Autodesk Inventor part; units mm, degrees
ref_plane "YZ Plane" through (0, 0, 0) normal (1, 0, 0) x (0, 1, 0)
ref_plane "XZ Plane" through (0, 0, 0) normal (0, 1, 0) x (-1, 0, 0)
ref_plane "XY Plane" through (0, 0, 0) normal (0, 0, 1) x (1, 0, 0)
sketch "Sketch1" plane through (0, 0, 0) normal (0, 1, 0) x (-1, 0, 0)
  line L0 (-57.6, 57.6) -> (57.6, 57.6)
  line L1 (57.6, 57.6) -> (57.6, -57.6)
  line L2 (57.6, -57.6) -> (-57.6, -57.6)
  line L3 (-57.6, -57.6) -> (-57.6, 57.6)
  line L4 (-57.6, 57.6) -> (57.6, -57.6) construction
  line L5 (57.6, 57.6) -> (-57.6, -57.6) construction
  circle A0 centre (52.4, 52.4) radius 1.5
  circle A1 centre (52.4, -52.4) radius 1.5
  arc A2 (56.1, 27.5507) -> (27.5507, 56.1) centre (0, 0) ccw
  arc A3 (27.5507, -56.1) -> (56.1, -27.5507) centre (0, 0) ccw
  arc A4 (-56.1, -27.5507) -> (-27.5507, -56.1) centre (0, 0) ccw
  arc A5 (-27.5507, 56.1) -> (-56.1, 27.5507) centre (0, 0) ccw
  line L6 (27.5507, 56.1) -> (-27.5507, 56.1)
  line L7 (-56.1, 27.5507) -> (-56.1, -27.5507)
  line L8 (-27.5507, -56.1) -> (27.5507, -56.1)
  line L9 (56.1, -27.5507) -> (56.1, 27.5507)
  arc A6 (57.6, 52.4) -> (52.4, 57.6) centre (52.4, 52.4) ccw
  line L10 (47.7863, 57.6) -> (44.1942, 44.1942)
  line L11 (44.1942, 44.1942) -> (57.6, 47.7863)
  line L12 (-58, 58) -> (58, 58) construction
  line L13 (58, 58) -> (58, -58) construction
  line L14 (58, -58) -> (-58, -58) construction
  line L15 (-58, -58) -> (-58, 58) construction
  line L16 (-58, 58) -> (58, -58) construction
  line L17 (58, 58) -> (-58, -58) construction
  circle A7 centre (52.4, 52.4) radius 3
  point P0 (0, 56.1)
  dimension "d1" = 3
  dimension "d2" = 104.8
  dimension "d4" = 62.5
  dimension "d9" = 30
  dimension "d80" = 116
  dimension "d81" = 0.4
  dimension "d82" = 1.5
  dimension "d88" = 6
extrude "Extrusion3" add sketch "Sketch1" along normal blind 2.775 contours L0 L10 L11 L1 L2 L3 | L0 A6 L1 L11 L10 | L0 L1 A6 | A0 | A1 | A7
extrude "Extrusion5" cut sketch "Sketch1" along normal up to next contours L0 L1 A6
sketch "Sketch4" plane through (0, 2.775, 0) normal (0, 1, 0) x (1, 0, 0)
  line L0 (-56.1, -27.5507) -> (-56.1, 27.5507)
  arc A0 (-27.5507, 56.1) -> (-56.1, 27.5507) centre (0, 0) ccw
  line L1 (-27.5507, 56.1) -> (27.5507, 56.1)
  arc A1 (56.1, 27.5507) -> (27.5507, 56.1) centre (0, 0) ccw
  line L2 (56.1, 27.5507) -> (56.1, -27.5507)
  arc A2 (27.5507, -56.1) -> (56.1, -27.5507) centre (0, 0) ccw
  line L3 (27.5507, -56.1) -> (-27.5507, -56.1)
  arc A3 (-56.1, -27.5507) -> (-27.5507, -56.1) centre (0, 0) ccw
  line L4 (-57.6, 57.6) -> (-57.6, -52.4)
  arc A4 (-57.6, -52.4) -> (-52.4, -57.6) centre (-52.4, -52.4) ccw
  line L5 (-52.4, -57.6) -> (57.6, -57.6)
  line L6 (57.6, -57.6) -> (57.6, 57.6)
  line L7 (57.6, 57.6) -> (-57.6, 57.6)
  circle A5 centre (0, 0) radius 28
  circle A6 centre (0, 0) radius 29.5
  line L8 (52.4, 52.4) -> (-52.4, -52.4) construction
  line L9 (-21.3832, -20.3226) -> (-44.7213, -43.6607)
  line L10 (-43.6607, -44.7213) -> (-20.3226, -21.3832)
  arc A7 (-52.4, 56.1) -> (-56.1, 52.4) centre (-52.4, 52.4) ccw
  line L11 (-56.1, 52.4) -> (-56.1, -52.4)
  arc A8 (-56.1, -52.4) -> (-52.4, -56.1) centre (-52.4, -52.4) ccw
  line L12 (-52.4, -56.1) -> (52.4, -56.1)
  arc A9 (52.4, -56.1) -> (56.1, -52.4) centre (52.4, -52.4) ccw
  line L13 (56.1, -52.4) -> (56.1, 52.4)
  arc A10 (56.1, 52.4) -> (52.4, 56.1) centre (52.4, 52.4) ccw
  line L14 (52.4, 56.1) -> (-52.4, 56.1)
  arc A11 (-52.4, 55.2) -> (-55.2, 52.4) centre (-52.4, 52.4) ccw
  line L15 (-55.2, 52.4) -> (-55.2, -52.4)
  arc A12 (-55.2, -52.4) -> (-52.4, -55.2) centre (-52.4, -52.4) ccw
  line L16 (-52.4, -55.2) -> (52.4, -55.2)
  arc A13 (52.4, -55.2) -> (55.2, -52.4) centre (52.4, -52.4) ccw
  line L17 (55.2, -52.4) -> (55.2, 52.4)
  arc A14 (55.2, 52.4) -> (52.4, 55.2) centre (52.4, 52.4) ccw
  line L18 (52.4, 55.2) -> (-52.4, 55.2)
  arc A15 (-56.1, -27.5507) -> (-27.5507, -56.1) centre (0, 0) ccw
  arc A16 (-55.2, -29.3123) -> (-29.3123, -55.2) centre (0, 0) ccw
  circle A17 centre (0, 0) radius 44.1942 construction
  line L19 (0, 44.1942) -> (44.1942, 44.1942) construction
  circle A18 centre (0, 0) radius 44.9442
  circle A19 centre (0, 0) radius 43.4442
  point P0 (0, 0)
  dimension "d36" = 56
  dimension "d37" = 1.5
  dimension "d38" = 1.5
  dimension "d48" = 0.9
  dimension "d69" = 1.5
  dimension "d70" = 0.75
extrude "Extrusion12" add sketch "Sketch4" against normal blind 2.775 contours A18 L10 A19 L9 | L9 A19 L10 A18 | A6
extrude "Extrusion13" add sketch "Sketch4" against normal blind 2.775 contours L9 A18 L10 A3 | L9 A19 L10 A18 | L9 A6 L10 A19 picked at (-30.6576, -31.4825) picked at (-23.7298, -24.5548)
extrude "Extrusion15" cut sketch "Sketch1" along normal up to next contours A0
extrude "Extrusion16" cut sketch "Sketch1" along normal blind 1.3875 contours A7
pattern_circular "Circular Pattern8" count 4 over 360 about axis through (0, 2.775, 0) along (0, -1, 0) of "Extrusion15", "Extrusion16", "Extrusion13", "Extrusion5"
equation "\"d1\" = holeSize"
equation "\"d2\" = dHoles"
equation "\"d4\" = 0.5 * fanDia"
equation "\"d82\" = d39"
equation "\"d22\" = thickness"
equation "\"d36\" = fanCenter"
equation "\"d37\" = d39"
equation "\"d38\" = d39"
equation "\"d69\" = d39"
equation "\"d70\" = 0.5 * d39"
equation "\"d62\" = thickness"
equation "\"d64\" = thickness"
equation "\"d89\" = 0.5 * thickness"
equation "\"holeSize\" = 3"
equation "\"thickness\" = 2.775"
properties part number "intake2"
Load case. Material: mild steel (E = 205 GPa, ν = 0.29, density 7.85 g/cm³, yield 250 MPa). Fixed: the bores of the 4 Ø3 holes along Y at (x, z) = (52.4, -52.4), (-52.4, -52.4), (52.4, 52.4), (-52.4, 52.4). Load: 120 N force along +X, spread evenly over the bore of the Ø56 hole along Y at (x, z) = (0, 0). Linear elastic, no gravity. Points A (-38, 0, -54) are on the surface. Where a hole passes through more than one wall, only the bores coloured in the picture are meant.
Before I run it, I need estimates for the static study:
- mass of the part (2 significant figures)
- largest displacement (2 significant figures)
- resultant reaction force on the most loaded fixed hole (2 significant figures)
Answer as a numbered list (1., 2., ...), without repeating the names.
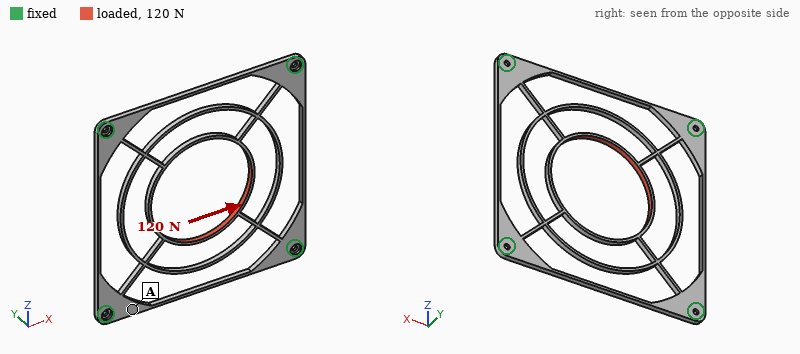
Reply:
1. 60 g
2. 0.18 mm
3. 39 N
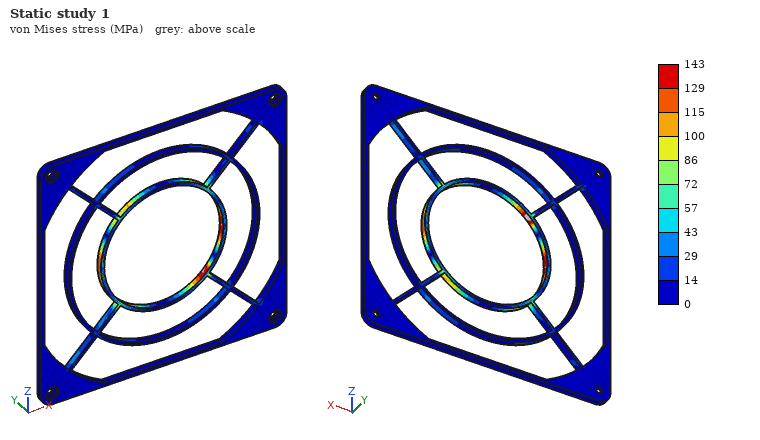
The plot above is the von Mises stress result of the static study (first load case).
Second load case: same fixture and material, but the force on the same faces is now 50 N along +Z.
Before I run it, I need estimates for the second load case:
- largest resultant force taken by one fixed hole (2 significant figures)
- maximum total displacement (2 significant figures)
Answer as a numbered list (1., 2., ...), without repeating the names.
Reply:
1. 16 N
2. 73 µm
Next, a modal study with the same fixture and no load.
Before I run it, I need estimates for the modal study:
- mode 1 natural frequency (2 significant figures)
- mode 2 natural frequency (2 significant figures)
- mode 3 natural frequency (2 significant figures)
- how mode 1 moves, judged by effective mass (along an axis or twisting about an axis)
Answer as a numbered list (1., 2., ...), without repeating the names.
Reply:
1. 820 Hz
2. 1100 Hz
3. 1100 Hz
4. along Y
